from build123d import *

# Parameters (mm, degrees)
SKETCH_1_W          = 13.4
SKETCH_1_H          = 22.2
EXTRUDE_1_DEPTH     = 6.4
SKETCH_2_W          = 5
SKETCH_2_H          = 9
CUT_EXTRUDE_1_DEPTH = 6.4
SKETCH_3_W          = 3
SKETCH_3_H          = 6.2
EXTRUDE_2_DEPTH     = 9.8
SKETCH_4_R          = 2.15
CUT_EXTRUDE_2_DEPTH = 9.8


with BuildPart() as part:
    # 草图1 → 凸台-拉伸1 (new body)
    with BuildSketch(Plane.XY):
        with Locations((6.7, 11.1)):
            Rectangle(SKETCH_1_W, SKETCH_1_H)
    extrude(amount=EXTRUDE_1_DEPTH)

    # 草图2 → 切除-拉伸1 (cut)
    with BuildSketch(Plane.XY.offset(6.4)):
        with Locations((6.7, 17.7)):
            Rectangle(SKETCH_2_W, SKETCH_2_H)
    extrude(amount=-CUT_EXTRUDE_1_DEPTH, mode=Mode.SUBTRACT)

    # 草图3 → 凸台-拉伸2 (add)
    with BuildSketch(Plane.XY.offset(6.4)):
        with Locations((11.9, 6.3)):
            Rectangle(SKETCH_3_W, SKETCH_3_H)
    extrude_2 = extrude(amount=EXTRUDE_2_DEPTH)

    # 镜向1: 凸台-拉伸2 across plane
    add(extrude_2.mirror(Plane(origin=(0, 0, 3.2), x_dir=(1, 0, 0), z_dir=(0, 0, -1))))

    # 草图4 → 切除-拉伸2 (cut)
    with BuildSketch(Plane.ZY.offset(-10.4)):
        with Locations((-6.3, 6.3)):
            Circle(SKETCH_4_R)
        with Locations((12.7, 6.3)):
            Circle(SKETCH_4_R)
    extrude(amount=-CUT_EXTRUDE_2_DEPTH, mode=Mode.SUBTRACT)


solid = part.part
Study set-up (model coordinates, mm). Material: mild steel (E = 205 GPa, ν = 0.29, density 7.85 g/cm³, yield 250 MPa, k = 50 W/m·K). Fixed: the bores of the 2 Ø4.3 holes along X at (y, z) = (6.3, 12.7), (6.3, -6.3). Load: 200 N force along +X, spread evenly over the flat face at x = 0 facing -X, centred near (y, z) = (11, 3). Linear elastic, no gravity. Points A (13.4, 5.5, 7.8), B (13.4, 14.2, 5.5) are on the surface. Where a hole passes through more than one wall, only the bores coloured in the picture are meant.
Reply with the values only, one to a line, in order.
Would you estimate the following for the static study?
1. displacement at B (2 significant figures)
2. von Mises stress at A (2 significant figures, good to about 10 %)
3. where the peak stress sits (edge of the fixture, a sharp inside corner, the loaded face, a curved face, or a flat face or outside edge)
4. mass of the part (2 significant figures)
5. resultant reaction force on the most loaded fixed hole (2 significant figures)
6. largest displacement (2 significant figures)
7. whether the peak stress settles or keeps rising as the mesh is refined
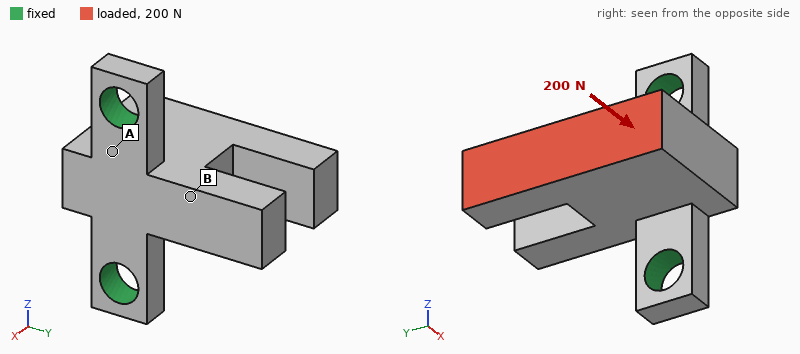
6.8 µm
42 MPa
edge of the fixture
15 g
100 N
18 µm
keeps rising
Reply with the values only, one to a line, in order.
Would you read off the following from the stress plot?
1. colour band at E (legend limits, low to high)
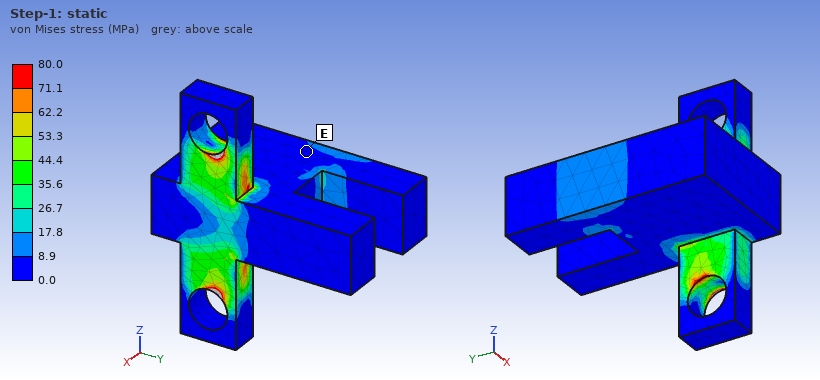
0.0 to 8.9 MPa
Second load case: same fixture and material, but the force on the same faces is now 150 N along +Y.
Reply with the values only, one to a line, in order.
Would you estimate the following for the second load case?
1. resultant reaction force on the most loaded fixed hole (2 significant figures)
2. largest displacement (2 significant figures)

75 N
28 µm
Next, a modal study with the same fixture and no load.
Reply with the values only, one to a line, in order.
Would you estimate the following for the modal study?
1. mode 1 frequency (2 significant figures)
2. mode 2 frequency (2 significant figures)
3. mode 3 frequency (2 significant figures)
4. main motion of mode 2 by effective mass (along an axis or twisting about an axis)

5200 Hz
12 kHz
19 kHz
along Z
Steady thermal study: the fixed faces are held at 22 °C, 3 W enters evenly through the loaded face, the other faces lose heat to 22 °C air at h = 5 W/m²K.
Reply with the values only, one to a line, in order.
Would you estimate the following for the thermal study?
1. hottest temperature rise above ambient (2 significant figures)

22 K
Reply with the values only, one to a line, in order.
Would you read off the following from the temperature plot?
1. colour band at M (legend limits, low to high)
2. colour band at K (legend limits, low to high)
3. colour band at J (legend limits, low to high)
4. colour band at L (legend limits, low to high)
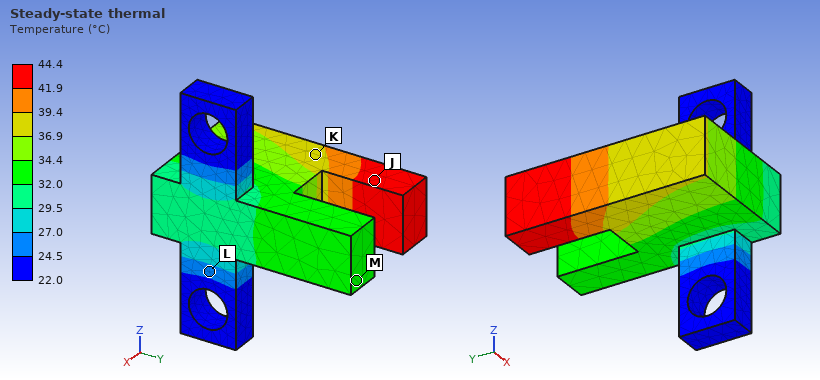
32.0 to 34.4 °C
36.9 to 39.4 °C
41.9 to 44.4 °C
24.5 to 27.0 °C
